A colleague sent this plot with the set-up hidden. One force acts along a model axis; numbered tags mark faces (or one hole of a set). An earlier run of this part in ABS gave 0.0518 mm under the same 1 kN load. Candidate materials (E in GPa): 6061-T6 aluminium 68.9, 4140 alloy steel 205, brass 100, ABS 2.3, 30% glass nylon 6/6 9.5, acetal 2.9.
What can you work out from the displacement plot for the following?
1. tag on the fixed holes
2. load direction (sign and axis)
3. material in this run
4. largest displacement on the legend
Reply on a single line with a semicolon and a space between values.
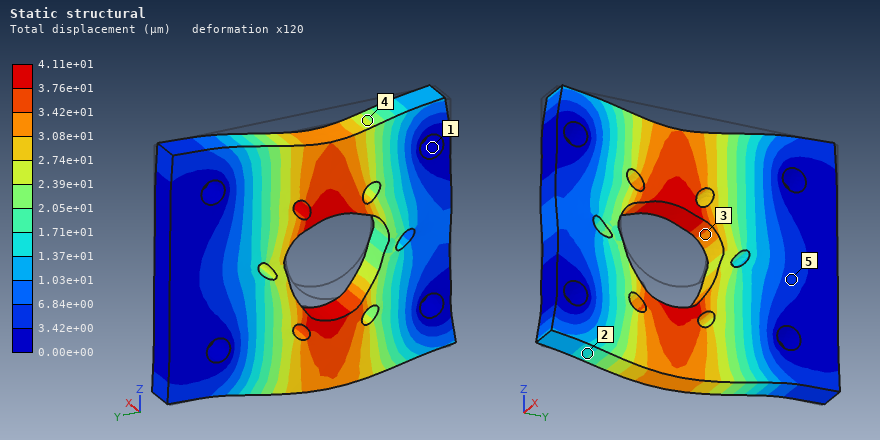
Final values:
1; -Z; acetal; 4.11e+01 µm
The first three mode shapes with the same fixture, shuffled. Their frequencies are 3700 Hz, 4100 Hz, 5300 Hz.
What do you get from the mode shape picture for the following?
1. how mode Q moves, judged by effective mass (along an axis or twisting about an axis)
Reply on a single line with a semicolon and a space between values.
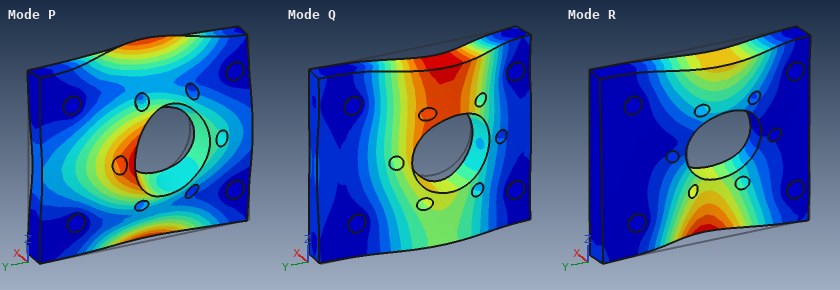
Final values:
along X
